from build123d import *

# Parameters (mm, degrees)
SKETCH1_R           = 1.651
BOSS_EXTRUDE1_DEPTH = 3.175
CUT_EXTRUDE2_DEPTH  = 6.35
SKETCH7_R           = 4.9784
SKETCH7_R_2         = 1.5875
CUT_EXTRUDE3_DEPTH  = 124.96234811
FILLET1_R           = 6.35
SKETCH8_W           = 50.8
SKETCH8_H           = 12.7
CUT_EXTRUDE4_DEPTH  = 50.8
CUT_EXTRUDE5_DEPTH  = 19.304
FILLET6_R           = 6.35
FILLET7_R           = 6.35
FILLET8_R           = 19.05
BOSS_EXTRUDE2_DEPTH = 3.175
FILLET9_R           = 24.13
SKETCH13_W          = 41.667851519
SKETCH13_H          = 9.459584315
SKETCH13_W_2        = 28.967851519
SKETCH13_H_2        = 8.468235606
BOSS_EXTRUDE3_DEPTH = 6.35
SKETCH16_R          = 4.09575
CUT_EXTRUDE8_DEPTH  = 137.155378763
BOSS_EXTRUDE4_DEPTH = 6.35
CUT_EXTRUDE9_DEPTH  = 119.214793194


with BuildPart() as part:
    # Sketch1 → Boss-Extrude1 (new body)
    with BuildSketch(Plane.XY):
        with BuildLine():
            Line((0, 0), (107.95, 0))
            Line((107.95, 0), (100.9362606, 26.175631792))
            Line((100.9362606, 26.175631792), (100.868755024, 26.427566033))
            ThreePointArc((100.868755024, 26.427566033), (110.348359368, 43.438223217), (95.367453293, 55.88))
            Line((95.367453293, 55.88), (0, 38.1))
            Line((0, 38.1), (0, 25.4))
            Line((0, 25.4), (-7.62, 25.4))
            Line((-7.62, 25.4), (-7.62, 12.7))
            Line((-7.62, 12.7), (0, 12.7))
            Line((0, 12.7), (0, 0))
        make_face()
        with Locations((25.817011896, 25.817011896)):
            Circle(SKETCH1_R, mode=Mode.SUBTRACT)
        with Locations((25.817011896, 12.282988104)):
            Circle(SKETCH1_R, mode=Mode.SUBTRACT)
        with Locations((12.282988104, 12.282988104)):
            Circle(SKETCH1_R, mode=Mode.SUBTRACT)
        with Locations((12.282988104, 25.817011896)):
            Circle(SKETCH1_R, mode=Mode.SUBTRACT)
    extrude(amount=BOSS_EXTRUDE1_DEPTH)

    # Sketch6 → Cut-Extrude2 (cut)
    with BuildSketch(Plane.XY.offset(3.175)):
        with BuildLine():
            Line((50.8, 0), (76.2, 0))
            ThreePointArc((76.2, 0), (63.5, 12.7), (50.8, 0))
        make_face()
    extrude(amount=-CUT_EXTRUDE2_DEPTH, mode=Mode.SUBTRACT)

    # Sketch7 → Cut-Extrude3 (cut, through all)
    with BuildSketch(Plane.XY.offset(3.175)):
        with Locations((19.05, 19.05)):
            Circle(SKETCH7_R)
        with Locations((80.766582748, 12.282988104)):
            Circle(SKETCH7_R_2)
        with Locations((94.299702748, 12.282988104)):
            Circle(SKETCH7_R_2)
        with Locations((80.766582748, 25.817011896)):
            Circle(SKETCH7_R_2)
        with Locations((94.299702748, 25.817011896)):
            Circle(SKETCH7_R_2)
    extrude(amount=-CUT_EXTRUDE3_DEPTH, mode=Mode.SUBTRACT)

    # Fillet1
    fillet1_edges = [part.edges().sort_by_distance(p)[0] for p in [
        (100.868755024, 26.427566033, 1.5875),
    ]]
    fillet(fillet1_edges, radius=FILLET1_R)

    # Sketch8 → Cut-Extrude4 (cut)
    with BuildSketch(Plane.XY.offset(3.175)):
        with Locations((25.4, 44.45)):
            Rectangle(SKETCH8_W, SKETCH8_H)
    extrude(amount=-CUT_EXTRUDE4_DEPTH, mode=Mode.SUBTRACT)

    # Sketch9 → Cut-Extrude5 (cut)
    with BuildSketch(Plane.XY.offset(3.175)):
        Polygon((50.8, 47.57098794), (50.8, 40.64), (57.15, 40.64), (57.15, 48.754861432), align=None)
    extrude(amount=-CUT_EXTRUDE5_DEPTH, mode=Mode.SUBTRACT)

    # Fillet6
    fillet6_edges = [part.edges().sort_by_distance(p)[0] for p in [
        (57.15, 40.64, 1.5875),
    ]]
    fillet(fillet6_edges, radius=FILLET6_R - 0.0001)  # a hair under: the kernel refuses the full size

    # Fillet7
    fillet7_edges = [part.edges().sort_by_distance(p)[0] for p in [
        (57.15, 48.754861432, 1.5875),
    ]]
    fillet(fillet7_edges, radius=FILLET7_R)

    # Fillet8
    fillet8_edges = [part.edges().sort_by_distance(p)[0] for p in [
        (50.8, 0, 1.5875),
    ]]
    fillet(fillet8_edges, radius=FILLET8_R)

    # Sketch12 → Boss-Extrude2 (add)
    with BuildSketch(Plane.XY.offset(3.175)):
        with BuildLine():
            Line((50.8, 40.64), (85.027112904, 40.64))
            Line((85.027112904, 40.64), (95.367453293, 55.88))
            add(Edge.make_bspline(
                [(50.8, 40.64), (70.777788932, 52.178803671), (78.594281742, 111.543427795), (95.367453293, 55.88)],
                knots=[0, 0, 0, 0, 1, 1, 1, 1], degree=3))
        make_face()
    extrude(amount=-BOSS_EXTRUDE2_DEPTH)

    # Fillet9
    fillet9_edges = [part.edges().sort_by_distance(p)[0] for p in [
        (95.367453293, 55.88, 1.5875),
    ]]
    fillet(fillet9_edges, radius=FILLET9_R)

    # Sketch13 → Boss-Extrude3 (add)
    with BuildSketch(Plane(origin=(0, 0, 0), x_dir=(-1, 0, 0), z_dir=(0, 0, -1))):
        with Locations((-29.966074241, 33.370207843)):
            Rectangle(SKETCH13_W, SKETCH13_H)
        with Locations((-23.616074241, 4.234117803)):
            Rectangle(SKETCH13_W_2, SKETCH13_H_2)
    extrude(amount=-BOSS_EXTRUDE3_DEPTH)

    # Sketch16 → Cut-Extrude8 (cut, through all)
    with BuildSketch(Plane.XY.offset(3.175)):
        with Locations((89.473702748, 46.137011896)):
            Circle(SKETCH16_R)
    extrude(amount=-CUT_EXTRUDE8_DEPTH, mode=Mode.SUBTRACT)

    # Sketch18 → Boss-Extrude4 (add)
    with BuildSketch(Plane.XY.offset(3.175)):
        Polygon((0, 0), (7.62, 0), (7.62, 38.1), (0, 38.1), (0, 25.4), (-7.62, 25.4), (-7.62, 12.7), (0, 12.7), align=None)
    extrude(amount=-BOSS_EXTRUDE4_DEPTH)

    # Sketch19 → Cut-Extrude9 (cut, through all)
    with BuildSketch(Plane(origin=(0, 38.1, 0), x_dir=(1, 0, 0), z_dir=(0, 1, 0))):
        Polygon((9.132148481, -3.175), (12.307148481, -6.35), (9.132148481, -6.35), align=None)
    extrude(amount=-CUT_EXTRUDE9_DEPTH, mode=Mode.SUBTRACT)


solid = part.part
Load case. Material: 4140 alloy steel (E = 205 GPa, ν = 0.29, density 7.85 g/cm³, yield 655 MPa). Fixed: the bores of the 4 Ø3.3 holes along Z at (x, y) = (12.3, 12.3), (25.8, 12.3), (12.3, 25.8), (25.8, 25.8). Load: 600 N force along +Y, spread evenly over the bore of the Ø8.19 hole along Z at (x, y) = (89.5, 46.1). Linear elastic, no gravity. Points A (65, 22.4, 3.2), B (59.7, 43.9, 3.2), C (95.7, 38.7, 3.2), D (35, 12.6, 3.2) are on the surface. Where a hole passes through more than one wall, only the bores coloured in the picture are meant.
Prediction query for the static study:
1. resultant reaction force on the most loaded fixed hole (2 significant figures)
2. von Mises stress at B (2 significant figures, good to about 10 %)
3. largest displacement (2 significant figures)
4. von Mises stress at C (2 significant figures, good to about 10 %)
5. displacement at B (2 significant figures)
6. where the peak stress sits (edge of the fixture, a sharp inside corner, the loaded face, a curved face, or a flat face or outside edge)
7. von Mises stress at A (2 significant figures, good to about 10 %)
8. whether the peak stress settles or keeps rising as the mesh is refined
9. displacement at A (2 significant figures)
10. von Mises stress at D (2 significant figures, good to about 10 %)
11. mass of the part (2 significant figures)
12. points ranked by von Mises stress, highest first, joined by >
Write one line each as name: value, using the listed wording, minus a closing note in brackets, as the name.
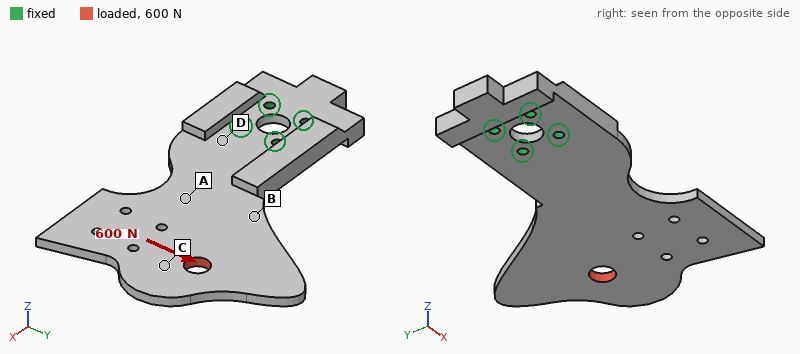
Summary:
resultant reaction force on the most loaded fixed hole: 1.4 kN
von Mises stress at B: 13 MPa
largest displacement: 69 µm
von Mises stress at C: 6.9 MPa
displacement at B: 26 µm
where the peak stress sits: edge of the fixture
von Mises stress at A: 23 MPa
whether the peak stress settles or keeps rising as the mesh is refined: keeps rising
displacement at A: 21 µm
von Mises stress at D: 37 MPa
mass of the part: 150 g
points ranked by von Mises stress, highest first, joined by >: D > A > B > C
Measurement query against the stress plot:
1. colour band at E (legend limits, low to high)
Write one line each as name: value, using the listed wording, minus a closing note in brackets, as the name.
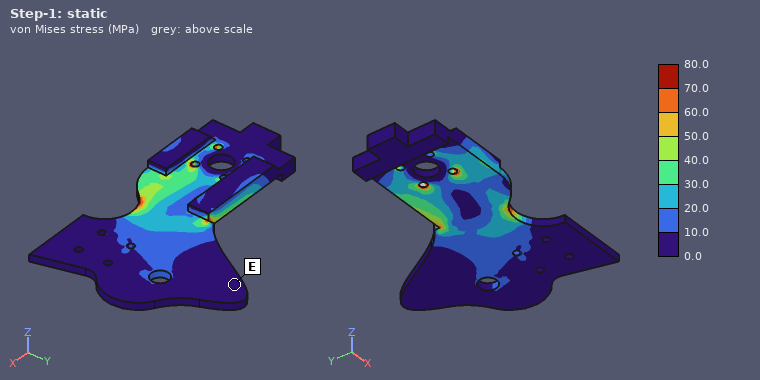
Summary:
colour band at E: 0.0 to 10.0 MPa
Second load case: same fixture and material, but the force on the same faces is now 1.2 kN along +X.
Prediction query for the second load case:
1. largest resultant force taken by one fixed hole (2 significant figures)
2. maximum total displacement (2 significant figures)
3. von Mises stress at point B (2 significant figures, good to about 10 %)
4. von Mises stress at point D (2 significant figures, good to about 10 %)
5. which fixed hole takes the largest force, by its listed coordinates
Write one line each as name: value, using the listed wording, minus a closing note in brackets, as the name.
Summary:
largest resultant force taken by one fixed hole: 1.5 kN
maximum total displacement: 82 µm
von Mises stress at point B: 29 MPa
von Mises stress at point D: 22 MPa
which fixed hole takes the largest force, by its listed coordinates: (25.8, 25.8)
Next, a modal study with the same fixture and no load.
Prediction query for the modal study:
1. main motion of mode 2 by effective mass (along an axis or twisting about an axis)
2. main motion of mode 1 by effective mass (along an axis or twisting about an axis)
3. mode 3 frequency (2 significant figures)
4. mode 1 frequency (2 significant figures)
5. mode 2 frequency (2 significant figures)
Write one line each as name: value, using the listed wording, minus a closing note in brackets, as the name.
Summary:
main motion of mode 2 by effective mass: twisting about X
main motion of mode 1 by effective mass: along Z
mode 3 frequency: 2400 Hz
mode 1 frequency: 420 Hz
mode 2 frequency: 860 Hz
